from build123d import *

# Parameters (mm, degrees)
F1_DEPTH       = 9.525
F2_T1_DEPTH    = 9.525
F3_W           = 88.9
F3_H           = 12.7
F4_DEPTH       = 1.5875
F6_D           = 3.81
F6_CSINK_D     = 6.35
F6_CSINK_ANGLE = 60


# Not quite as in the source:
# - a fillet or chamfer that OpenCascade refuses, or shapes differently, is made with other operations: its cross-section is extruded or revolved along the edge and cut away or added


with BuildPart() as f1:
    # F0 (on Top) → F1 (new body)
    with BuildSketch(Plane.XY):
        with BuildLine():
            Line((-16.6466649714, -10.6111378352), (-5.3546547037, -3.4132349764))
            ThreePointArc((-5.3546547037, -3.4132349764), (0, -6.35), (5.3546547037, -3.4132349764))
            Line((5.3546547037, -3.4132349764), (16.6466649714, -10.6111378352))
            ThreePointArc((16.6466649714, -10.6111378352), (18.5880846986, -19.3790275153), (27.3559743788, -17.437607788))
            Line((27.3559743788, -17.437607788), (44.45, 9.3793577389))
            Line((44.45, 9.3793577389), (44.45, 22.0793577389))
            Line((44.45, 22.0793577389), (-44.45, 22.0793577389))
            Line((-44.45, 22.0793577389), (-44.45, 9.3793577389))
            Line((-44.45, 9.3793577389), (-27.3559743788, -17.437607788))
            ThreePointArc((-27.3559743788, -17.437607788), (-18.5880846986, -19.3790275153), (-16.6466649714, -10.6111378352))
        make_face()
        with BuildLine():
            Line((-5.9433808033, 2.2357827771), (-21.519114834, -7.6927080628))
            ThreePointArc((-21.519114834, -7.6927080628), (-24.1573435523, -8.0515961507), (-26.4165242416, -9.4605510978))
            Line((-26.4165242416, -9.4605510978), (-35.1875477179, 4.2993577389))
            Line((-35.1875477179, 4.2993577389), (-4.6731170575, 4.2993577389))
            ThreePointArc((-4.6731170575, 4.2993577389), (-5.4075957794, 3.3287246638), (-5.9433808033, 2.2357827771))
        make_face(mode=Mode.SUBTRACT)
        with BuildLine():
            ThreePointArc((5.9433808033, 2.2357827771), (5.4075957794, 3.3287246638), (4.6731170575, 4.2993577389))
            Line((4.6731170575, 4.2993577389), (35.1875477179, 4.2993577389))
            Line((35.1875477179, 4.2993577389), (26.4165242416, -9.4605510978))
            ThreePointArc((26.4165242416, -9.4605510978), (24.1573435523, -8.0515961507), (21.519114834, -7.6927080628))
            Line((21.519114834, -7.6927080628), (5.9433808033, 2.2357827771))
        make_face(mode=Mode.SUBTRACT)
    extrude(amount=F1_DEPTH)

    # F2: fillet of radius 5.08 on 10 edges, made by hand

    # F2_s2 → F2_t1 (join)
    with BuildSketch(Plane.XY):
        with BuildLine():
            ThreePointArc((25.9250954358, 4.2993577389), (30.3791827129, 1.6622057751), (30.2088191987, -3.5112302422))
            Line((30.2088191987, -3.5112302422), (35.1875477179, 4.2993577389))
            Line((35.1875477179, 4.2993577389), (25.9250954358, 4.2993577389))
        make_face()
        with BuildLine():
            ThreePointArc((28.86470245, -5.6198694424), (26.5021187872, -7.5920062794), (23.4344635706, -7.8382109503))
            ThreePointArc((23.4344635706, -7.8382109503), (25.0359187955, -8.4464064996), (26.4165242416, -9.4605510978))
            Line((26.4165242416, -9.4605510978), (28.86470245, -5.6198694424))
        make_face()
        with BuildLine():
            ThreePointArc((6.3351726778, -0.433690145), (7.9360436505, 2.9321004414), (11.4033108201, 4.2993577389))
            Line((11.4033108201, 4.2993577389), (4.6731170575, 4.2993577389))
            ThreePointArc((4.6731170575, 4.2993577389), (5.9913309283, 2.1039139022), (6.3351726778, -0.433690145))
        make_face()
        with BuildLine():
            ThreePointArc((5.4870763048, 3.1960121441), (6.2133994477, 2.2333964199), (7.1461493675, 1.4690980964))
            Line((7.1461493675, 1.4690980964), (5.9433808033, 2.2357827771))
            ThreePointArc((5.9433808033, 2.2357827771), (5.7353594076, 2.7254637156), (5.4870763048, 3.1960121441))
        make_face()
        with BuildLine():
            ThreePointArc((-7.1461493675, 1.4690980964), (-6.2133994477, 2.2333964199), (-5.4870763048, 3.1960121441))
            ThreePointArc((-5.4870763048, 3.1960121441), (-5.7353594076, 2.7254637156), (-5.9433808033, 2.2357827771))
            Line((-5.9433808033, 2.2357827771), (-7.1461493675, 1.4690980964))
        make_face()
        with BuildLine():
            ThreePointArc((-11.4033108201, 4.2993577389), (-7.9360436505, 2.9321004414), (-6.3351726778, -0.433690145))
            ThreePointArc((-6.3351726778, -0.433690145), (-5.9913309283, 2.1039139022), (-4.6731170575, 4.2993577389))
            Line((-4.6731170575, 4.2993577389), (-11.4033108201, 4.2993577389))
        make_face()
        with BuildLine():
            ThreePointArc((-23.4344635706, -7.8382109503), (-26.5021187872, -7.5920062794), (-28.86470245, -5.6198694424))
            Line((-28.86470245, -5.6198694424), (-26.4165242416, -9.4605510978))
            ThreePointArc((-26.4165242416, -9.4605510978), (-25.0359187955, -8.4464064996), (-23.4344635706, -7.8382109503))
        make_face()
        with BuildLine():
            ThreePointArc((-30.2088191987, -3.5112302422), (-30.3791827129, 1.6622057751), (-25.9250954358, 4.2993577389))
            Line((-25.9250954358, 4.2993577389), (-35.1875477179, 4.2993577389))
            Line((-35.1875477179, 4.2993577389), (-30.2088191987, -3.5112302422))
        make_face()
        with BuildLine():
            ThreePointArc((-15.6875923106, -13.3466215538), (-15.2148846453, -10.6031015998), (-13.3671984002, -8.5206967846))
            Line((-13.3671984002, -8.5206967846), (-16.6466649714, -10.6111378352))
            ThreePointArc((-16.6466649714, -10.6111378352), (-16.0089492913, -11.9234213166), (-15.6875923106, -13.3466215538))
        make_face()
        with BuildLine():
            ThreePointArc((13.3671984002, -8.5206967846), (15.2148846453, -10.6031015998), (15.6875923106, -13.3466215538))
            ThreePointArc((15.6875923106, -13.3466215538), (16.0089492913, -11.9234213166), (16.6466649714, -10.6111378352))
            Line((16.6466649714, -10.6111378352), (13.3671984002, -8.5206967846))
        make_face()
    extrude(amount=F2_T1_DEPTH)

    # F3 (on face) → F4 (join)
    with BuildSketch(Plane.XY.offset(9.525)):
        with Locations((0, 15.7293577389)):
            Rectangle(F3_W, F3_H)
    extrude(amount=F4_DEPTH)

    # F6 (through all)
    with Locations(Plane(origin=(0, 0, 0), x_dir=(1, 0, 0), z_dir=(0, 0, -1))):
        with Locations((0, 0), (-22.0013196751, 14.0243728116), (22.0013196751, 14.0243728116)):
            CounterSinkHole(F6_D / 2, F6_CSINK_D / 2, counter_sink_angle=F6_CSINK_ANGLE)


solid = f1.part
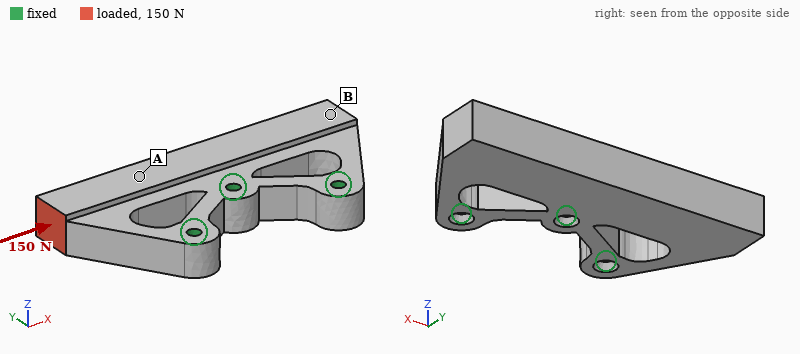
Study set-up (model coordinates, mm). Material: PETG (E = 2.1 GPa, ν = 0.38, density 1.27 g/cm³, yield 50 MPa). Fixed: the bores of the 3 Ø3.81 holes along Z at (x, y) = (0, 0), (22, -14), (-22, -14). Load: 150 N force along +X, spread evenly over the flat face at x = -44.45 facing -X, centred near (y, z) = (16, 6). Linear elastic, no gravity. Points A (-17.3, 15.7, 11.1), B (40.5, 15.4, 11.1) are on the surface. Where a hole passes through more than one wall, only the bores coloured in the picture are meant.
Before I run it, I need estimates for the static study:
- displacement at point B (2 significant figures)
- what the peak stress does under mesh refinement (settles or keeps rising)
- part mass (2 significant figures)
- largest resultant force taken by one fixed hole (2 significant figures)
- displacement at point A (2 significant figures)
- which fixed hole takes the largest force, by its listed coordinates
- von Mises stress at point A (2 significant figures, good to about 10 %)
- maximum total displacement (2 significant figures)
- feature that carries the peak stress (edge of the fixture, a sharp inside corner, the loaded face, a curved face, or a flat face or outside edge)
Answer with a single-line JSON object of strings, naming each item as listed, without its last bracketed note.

{"displacement at point B": "29 µm", "what the peak stress does under mesh refinement": "keeps rising", "part mass": "30 g", "largest resultant force taken by one fixed hole": "150 N", "displacement at point A": "33 µm", "which fixed hole takes the largest force, by its listed coordinates": "(0, 0)", "von Mises stress at point A": "0.80 MPa", "maximum total displacement": "60 µm", "feature that carries the peak stress": "edge of the fixture"}
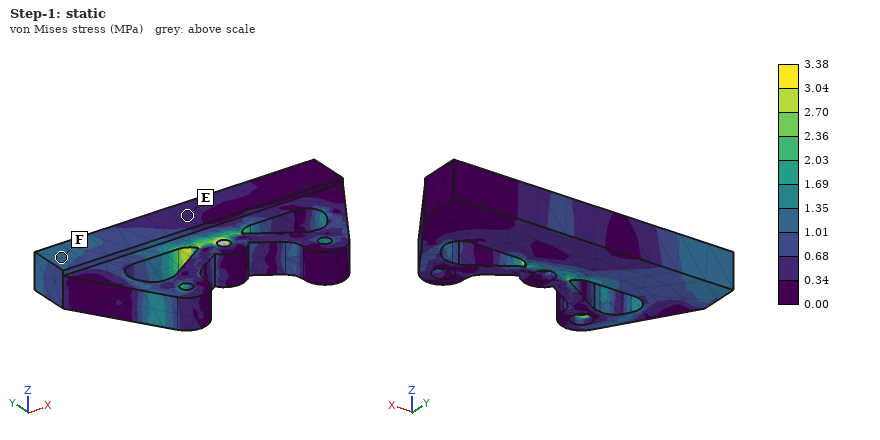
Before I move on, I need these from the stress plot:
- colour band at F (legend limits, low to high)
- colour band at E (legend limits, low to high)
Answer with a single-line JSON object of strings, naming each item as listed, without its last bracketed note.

{"colour band at F": "1.01 to 1.35 MPa", "colour band at E": "0.34 to 0.68 MPa"}
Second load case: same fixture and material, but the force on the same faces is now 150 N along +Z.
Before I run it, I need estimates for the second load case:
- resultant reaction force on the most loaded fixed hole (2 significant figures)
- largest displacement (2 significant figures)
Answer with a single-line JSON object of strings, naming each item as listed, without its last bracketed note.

{"resultant reaction force on the most loaded fixed hole": "110 N", "largest displacement": "1.1 mm"}
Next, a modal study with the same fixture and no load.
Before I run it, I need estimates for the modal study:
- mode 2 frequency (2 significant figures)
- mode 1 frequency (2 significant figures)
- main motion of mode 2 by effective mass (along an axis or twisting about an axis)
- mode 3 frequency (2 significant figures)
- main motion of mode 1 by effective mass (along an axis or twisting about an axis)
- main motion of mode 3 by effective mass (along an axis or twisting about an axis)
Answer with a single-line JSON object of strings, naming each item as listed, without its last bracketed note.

{"mode 2 frequency": "1100 Hz", "mode 1 frequency": "1000 Hz", "main motion of mode 2 by effective mass": "along Z", "mode 3 frequency": "2100 Hz", "main motion of mode 1 by effective mass": "twisting about Y", "main motion of mode 3 by effective mass": "along X"}
